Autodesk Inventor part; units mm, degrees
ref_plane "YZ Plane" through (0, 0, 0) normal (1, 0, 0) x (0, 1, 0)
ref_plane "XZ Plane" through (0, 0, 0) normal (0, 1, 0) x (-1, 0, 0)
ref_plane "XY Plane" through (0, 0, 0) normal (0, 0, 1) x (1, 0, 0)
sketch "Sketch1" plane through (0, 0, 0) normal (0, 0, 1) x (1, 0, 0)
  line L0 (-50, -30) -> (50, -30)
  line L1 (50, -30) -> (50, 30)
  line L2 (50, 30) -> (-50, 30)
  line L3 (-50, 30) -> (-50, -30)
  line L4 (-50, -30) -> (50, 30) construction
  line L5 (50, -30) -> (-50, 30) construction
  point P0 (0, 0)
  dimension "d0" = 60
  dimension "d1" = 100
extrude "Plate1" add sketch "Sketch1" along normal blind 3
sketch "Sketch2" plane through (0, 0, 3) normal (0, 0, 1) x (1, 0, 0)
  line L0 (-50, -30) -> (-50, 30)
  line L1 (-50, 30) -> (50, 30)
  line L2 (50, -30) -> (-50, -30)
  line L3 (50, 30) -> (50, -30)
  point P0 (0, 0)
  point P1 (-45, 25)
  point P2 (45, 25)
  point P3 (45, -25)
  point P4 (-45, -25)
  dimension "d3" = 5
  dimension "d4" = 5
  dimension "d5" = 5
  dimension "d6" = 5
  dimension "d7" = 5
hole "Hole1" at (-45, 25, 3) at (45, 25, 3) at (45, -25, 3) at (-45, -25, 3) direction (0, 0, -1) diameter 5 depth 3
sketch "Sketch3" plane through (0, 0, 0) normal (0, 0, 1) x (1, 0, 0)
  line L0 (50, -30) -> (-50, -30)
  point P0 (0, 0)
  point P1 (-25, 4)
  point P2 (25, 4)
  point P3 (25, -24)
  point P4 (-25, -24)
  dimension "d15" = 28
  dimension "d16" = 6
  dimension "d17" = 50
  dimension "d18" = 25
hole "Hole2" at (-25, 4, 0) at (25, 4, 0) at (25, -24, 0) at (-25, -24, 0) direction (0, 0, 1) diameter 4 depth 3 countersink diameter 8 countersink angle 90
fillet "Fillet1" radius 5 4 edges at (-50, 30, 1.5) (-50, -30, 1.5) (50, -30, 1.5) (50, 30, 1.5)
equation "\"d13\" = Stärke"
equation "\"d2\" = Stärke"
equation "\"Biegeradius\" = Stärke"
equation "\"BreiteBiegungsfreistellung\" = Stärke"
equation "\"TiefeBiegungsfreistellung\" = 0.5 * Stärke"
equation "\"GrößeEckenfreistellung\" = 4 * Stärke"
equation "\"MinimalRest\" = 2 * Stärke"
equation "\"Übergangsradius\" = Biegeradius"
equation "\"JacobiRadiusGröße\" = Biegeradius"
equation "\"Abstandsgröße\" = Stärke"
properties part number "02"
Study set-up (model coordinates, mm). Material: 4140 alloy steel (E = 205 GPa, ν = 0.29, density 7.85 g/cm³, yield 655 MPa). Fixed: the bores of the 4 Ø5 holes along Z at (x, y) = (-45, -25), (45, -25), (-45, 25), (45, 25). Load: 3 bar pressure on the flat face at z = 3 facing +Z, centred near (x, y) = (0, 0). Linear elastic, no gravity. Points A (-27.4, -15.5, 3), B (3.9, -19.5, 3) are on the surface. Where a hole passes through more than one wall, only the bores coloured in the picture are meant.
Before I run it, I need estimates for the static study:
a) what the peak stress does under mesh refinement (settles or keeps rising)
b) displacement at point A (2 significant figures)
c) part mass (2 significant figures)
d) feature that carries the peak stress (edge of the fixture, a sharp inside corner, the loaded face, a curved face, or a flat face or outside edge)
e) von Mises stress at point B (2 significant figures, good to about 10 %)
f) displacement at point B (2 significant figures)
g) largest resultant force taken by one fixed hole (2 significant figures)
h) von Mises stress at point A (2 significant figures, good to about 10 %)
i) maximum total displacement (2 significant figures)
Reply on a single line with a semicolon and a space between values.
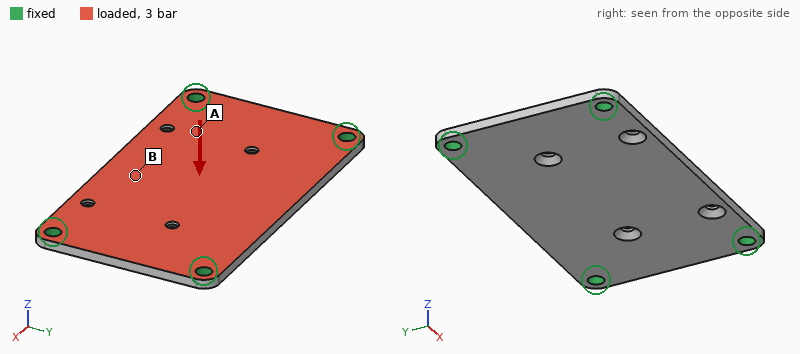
keeps rising; 0.064 mm; 140 g; edge of the fixture; 70 MPa; 0.13 mm; 440 N; 21 MPa; 0.14 mm
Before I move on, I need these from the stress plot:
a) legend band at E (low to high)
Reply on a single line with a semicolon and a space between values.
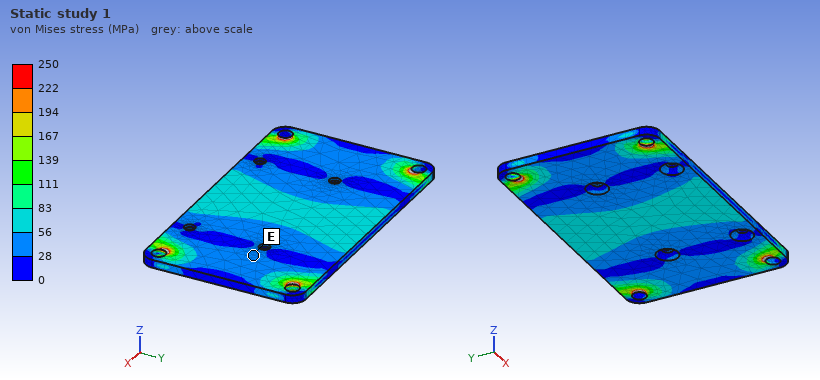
28 to 56 MPa
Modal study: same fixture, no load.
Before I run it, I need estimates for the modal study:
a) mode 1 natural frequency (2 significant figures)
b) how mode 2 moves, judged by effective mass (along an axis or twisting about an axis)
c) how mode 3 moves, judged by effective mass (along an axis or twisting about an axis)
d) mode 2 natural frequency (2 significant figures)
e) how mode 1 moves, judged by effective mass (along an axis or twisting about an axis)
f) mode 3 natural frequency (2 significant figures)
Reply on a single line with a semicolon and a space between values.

1700 Hz; twisting about X; twisting about Y; 2800 Hz; along Z; 4600 Hz
